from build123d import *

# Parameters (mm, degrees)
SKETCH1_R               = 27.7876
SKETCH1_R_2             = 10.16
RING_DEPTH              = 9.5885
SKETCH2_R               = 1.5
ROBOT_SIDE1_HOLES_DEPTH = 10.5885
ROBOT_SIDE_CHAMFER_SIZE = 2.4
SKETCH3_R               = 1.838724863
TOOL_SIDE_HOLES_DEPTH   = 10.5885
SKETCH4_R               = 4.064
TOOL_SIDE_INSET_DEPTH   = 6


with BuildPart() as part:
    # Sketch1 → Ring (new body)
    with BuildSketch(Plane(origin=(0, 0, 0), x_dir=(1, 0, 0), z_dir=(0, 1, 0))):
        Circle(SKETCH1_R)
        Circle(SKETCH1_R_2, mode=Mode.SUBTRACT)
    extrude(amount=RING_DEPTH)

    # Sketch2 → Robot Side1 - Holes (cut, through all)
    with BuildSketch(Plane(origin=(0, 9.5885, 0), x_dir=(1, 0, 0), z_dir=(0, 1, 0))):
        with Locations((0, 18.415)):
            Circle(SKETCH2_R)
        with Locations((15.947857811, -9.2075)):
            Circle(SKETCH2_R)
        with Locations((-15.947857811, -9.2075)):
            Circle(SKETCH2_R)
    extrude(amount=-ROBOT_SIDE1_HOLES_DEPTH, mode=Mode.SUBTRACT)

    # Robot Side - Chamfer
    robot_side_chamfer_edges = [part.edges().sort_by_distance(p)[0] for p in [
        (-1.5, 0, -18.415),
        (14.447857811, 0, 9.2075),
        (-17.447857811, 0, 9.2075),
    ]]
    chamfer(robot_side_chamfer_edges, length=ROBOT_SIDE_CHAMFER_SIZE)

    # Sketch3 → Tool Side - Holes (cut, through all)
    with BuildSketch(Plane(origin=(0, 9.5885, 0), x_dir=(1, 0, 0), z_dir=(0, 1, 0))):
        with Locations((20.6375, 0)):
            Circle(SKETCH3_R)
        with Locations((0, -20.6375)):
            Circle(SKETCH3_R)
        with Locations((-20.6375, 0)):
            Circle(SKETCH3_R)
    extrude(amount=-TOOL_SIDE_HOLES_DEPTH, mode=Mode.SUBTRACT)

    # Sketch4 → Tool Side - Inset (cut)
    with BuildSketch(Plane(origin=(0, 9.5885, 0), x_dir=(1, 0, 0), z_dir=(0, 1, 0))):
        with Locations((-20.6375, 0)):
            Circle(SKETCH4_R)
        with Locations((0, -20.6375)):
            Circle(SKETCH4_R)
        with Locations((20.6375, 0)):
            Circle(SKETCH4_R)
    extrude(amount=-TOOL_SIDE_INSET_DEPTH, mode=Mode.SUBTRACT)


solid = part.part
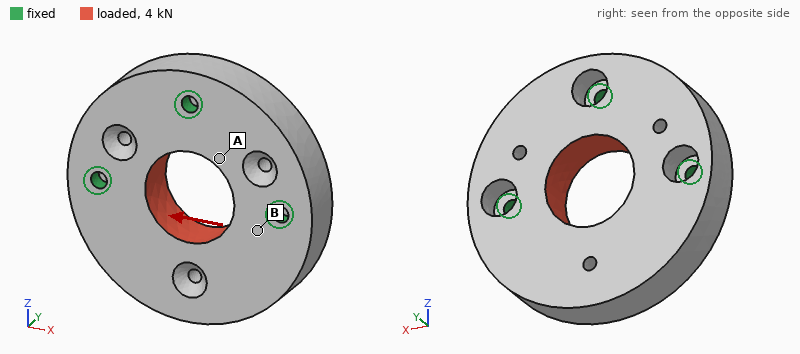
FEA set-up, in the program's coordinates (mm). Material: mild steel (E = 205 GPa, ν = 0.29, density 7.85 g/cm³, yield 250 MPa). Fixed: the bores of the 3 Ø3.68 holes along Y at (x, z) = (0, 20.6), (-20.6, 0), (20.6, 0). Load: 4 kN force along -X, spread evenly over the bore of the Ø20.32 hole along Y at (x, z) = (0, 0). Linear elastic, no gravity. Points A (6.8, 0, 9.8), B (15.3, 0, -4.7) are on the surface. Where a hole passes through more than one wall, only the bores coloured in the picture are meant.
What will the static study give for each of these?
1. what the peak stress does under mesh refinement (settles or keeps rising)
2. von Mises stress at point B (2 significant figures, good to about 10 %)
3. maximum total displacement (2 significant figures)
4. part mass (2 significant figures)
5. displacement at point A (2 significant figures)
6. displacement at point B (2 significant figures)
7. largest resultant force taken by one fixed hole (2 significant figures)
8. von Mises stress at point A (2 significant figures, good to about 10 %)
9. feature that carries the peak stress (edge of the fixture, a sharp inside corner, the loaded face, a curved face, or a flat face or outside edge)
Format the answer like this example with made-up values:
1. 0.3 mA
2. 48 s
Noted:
1. keeps rising
2. 24 MPa
3. 2.5 µm
4. 150 g
5. 1.00 µm
6. 1.1 µm
7. 1.6 kN
8. 11 MPa
9. edge of the fixture
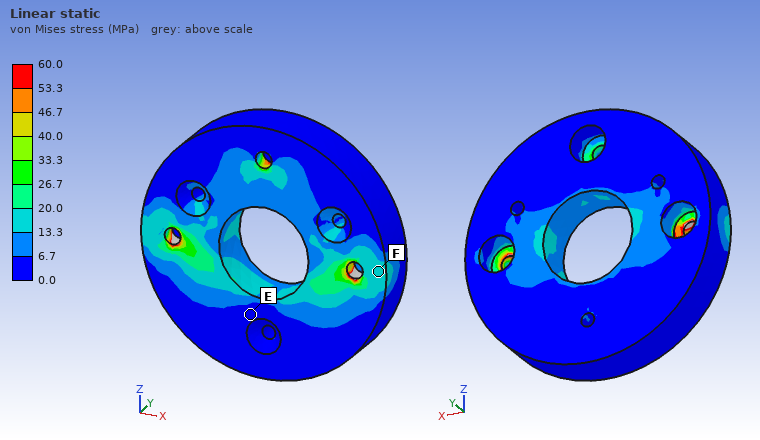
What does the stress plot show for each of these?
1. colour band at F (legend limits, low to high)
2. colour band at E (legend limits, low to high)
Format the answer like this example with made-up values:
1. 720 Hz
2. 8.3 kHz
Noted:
1. 13.3 to 20.0 MPa
2. 0.0 to 6.7 MPa
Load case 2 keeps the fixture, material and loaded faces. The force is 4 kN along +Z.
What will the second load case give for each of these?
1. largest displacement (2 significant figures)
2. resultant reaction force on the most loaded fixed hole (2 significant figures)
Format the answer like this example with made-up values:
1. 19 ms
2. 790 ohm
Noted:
1. 7.5 µm
2. 1.4 kN
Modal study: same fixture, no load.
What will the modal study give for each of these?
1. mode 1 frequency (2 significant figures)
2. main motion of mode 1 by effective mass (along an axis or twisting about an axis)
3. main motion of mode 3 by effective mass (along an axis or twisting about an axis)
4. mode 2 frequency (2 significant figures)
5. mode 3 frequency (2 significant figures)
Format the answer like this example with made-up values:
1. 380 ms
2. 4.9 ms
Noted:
1. 5700 Hz
2. along Y
3. along X
4. 14 kHz
5. 18 kHz
